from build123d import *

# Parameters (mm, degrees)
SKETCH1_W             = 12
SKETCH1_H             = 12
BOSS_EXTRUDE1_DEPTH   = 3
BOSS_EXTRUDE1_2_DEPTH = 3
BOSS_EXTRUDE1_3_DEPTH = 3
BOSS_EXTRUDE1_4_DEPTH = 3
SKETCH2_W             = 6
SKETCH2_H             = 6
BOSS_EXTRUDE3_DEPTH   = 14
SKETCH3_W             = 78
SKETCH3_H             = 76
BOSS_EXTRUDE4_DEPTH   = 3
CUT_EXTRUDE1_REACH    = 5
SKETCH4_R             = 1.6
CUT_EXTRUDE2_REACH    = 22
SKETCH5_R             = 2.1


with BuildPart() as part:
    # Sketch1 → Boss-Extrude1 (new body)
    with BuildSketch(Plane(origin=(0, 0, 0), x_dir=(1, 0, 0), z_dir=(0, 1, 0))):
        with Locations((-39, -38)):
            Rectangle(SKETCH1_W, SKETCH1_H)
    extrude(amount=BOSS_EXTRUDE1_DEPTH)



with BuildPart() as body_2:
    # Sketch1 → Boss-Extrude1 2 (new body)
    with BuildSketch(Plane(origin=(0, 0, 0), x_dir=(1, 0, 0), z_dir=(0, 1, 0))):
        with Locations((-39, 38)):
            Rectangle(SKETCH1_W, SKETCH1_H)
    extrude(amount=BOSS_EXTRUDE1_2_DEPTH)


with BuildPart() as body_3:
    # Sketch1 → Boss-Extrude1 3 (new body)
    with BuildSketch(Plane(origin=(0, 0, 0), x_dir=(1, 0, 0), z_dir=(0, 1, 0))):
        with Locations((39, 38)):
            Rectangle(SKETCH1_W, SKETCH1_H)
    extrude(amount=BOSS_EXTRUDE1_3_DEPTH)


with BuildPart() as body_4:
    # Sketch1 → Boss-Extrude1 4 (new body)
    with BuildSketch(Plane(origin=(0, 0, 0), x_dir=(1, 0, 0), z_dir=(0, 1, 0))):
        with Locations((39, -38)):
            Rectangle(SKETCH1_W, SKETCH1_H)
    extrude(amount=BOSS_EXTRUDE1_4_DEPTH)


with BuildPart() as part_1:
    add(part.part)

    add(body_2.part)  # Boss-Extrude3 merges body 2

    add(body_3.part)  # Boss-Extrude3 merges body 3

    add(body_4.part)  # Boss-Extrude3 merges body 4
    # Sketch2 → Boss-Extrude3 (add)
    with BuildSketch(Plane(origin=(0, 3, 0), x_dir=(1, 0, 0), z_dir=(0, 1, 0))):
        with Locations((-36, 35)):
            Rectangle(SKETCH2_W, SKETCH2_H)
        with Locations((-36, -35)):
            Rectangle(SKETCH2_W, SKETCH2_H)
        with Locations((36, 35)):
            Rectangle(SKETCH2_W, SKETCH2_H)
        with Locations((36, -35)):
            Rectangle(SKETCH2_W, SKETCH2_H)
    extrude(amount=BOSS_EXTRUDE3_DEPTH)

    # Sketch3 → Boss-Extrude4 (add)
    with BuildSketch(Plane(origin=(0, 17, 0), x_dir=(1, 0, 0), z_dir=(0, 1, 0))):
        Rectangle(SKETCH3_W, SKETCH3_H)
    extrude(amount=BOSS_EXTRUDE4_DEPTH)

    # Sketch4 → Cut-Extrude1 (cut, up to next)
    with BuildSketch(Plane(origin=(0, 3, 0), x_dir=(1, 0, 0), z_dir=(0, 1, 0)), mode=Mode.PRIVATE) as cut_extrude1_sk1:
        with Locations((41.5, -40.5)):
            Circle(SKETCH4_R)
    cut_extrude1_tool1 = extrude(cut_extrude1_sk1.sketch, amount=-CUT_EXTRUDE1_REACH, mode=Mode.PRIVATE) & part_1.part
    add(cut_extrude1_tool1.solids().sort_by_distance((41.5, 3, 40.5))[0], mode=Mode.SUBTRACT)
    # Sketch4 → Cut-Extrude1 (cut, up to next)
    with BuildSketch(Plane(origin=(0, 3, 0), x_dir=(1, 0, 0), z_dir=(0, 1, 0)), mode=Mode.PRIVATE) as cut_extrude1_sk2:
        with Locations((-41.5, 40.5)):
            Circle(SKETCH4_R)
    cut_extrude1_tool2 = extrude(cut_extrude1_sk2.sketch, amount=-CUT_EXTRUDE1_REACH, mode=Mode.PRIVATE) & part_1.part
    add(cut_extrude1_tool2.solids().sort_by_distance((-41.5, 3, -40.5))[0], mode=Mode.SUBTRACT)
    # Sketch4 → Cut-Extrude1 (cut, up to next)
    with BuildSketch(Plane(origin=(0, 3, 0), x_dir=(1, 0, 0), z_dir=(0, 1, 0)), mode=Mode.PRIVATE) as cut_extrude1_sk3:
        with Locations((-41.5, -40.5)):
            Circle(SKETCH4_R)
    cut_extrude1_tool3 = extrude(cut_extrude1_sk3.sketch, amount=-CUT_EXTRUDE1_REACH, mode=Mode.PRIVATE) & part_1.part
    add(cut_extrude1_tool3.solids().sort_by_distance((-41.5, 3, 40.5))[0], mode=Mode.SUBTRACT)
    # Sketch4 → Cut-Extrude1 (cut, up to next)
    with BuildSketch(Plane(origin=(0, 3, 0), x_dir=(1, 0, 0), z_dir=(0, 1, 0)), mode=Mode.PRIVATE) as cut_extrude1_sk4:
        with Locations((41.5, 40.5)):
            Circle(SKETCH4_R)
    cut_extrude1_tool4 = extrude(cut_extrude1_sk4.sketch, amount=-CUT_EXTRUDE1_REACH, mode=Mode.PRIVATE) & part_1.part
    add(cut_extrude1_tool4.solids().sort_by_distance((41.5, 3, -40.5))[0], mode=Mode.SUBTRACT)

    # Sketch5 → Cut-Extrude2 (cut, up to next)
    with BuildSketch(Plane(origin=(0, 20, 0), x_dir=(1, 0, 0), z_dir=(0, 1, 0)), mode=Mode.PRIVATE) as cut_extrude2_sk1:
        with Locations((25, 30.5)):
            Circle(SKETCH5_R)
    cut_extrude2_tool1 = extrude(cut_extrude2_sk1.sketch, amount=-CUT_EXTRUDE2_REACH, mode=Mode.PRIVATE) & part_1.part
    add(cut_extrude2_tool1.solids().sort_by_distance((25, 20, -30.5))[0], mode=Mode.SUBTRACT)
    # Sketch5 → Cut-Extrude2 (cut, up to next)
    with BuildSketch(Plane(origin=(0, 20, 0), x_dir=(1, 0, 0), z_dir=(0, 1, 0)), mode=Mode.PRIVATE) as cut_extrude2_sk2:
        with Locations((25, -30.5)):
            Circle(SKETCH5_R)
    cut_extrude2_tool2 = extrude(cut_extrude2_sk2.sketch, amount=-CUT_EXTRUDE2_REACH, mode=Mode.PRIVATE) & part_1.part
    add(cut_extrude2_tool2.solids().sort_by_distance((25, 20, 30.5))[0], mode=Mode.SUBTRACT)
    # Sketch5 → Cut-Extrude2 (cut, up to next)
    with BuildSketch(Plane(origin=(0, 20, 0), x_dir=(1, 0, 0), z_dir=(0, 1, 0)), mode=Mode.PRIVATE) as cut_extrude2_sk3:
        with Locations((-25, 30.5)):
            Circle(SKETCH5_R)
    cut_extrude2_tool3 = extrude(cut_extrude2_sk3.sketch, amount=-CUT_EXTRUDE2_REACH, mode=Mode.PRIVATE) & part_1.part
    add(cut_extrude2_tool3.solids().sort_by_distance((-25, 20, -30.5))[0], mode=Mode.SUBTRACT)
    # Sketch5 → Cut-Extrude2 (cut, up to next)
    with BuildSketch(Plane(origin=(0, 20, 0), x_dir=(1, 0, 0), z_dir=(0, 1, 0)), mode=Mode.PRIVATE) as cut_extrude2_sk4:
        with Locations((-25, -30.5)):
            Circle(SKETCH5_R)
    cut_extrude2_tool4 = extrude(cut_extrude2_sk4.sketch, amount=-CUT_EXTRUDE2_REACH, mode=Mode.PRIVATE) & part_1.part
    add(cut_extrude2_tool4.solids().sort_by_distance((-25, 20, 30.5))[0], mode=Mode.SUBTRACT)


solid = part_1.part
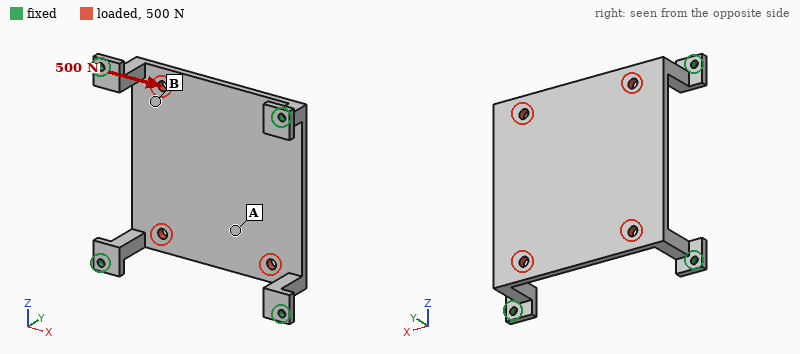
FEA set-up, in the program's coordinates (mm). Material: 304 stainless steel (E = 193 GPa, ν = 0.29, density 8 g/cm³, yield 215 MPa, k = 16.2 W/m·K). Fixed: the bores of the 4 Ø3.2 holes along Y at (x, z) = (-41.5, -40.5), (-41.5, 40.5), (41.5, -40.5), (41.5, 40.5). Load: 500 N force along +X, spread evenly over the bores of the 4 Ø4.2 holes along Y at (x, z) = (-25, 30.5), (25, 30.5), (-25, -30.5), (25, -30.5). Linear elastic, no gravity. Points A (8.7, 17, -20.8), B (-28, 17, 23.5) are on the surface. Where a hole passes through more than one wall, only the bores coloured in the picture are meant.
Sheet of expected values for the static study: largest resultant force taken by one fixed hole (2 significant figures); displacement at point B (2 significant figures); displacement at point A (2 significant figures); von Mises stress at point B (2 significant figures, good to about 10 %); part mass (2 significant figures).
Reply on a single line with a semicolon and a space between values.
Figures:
130 N; 23 µm; 24 µm; 16 MPa; 170 g
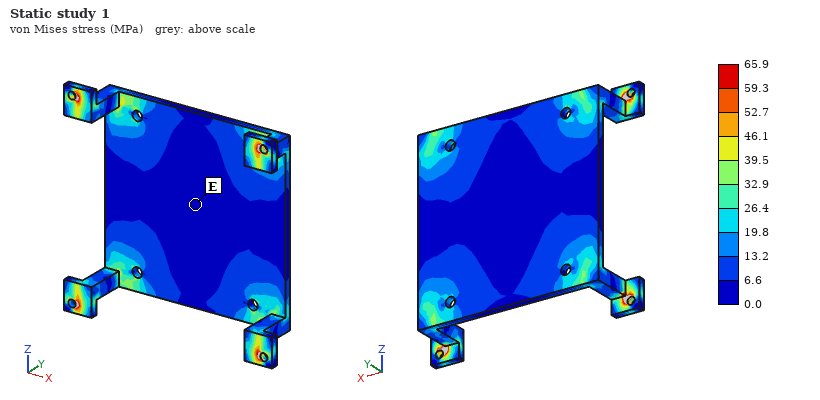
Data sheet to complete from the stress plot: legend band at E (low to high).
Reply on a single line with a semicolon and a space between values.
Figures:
0.0 to 6.6 MPa
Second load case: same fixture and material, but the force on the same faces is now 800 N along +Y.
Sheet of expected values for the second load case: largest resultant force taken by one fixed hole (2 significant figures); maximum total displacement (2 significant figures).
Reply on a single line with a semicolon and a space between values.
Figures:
250 N; 27 µm
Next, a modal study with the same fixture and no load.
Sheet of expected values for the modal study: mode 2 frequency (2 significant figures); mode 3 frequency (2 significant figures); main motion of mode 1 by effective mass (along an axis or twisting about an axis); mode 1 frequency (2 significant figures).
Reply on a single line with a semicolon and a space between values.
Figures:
1900 Hz; 1900 Hz; along Y; 1700 Hz
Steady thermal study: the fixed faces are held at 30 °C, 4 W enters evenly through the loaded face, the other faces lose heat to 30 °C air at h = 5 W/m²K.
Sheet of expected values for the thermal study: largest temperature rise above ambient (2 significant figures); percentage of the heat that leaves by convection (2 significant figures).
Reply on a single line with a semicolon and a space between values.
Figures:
33 K; 45 %
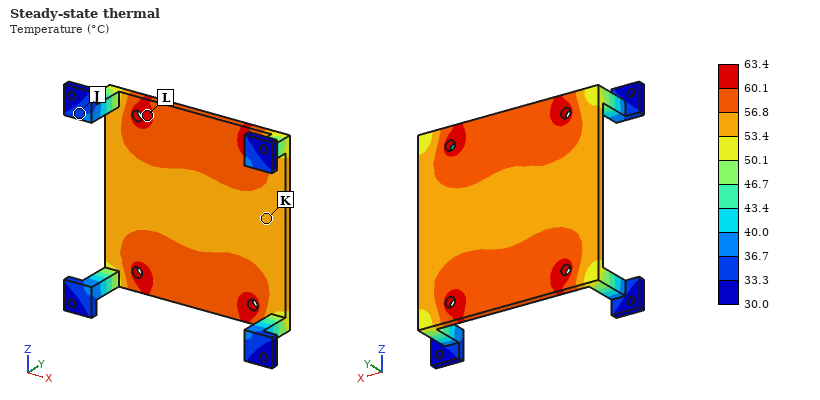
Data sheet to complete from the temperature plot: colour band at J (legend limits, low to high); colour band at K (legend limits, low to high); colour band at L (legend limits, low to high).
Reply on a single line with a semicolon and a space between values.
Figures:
33.3 to 36.7 °C; 53.4 to 56.8 °C; 60.1 to 63.4 °C
